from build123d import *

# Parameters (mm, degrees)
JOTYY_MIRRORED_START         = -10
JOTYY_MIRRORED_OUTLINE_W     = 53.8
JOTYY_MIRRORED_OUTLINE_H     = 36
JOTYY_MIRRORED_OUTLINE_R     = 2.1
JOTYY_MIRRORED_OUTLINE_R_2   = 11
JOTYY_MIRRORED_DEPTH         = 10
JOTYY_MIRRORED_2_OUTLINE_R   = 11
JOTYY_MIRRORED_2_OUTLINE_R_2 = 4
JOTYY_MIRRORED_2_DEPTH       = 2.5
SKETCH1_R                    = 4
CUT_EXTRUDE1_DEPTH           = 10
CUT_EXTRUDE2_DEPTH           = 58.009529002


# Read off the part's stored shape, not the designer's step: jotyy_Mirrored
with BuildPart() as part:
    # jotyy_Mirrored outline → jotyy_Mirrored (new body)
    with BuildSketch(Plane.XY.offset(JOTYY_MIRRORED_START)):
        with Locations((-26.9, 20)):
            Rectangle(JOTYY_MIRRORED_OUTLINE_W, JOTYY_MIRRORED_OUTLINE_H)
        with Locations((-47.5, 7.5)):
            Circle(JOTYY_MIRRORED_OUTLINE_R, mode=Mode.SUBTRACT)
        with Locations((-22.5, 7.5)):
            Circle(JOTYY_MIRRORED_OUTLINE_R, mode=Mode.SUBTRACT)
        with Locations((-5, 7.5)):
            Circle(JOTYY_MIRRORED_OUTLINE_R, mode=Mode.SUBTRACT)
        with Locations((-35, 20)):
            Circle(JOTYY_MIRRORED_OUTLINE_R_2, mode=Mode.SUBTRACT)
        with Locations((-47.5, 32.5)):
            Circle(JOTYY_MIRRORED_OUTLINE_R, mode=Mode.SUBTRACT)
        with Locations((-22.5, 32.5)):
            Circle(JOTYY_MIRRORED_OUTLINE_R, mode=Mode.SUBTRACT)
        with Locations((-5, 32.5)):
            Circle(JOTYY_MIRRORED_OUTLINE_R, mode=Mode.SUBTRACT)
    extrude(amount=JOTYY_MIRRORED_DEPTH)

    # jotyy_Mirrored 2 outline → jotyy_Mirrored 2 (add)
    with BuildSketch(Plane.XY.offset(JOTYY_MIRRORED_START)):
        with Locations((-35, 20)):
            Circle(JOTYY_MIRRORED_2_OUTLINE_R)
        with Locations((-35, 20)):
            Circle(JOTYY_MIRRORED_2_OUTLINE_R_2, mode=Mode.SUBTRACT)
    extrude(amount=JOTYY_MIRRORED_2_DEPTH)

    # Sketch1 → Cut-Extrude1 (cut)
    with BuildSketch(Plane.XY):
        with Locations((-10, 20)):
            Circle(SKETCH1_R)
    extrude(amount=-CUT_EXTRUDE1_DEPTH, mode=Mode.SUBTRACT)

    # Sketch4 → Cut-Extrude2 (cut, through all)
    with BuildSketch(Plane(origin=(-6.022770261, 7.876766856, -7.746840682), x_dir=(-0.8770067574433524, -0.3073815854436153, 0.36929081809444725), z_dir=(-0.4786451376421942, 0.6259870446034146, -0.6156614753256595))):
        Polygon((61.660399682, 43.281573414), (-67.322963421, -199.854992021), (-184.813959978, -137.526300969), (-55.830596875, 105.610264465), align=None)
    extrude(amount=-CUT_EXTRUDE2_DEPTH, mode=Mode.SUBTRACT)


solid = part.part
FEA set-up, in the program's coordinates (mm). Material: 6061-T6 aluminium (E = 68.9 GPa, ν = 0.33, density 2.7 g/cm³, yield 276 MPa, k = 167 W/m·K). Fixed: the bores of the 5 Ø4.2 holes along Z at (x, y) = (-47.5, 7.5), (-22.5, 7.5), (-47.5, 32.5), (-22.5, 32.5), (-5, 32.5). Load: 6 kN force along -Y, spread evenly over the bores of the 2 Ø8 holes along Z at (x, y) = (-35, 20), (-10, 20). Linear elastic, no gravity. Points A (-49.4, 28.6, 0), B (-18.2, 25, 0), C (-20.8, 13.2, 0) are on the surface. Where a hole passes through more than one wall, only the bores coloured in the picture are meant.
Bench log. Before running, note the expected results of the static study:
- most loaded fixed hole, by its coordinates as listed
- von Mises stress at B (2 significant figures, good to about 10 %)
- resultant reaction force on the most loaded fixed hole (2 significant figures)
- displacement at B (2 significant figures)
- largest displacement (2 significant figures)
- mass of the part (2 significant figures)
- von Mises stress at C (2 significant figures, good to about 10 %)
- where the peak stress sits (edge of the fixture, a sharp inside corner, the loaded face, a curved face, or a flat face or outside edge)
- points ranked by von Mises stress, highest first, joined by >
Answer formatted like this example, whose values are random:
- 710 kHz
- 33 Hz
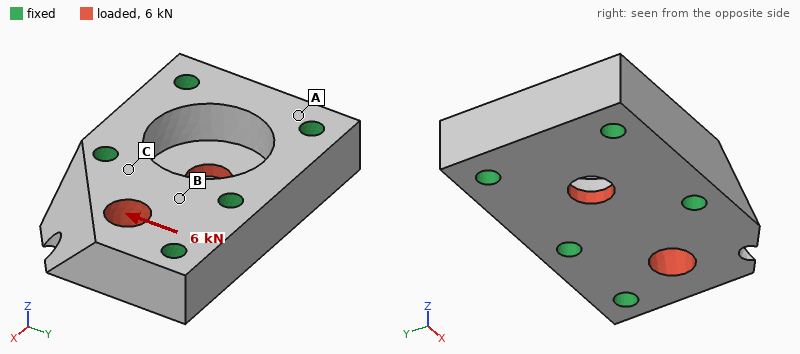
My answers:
- (-5, 32.5)
- 16 MPa
- 2.5 kN
- 1.6 µm
- 7.6 µm
- 38 g
- 10 MPa
- the loaded face
- B > C > A
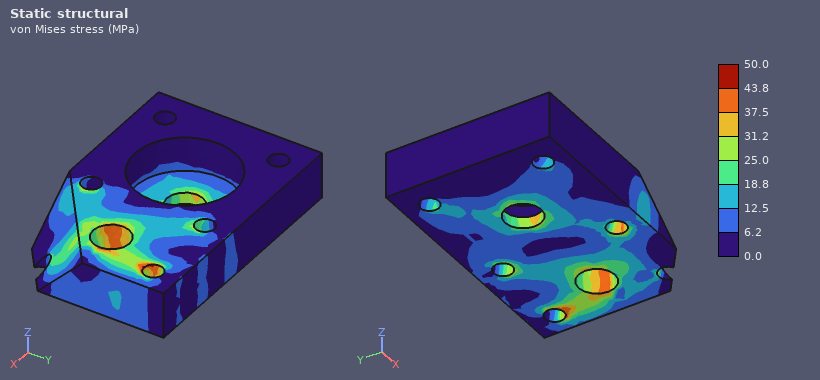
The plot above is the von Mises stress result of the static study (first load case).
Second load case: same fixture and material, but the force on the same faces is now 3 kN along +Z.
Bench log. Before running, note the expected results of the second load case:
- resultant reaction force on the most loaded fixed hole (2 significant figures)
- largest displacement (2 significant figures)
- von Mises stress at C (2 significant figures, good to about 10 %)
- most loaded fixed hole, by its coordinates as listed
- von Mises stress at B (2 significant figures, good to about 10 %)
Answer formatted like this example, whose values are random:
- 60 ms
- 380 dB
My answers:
- 1.2 kN
- 18 µm
- 14 MPa
- (-5, 32.5)
- 15 MPa
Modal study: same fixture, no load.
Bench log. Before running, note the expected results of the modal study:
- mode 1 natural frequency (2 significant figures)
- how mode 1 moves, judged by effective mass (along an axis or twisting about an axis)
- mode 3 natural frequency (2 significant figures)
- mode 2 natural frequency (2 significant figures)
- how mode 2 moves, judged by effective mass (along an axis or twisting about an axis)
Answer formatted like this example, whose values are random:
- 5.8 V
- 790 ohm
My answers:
- 28 kHz
- along Z
- 49 kHz
- 40 kHz
- along Z
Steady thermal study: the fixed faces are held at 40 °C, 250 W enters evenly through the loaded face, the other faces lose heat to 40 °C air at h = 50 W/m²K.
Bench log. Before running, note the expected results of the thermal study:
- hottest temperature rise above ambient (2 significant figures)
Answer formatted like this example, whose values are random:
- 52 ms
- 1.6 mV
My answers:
- 56 K
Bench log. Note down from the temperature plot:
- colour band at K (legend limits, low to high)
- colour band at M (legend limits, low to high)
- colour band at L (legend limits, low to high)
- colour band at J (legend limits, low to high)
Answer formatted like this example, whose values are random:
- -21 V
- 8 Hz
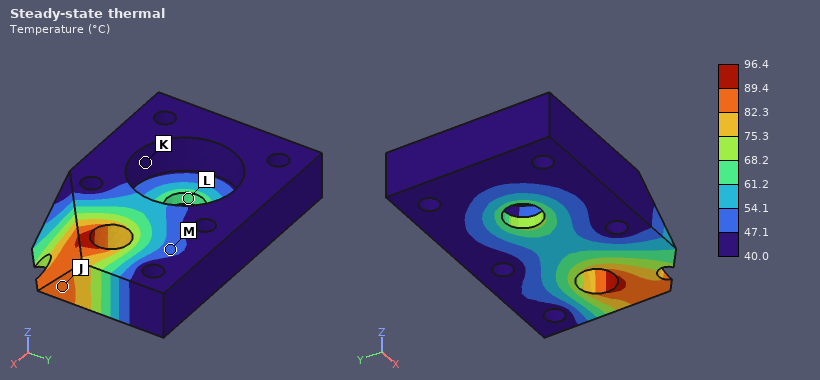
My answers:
- 40.0 to 47.1 °C
- 47.1 to 54.1 °C
- 61.2 to 68.2 °C
- 82.3 to 89.4 °C
